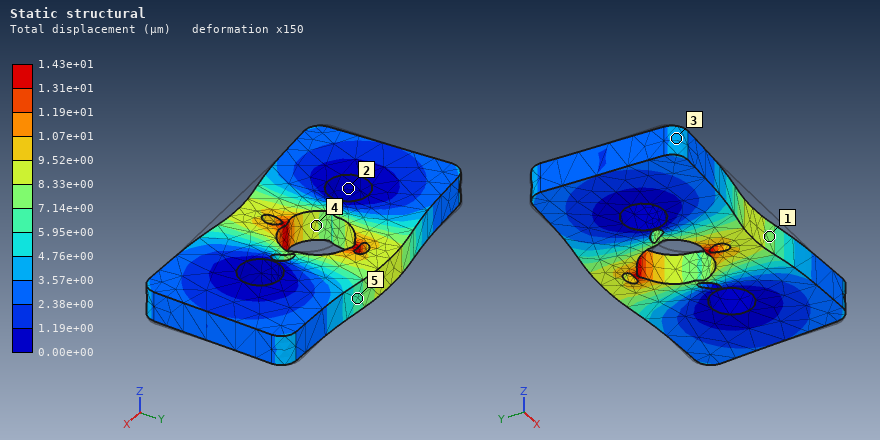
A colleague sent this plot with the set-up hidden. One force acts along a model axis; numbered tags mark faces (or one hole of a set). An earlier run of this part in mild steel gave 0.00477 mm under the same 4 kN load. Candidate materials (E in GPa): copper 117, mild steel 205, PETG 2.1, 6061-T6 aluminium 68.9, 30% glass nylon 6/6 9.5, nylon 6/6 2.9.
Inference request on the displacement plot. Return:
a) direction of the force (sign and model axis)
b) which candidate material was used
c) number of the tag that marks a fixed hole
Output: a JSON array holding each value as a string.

["+Y", "6061-T6 aluminium", "2"]
